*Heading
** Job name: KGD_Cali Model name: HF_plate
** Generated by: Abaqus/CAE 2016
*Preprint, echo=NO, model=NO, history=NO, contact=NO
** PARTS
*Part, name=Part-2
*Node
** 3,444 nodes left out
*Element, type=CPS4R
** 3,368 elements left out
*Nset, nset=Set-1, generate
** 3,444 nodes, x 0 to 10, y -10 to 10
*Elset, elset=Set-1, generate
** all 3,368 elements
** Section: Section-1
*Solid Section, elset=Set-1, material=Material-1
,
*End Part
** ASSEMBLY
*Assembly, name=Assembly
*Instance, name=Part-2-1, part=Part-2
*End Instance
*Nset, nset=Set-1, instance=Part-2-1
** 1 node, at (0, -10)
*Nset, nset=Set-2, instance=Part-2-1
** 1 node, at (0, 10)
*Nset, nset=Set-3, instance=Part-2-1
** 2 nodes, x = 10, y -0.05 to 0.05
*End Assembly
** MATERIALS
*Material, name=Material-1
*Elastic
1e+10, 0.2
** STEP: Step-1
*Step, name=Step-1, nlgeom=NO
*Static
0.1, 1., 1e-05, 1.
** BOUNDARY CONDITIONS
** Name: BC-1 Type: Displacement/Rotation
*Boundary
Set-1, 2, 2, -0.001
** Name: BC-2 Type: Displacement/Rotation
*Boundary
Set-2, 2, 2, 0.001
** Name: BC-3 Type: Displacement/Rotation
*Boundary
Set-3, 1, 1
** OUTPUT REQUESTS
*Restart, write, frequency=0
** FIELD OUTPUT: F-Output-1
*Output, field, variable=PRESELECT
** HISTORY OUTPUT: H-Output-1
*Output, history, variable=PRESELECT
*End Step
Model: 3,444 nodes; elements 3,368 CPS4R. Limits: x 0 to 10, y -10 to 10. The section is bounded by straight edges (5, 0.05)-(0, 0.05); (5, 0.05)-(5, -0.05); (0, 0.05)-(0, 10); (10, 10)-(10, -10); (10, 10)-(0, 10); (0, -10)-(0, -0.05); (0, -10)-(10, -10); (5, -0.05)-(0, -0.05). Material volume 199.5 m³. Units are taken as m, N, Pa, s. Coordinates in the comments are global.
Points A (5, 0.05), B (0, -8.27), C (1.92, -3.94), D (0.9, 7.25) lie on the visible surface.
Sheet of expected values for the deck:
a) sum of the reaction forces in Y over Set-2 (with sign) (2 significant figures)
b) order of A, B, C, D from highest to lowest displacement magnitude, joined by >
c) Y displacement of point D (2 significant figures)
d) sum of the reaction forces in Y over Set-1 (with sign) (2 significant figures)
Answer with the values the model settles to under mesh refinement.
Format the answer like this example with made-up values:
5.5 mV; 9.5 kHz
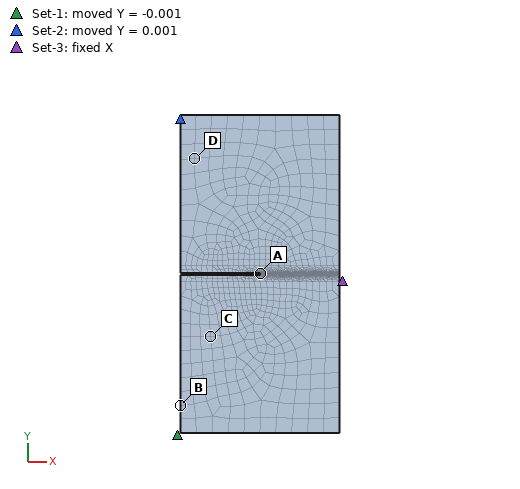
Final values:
4.3e+05 N; B > D > C > A; 6.1e-04 m; -4.3e+05 N
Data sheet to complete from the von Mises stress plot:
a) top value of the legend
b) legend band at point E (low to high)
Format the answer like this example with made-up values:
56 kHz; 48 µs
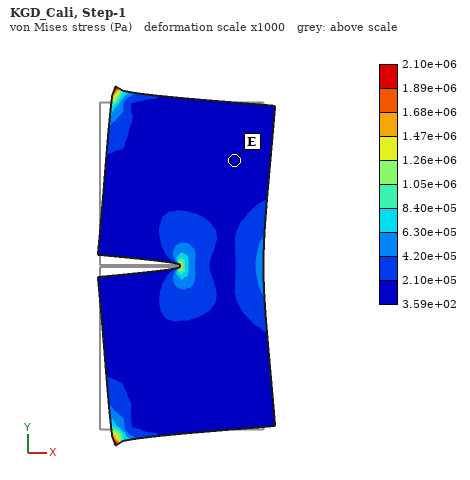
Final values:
2.10e+06 Pa; 3.59e+02 to 2.10e+05 Pa
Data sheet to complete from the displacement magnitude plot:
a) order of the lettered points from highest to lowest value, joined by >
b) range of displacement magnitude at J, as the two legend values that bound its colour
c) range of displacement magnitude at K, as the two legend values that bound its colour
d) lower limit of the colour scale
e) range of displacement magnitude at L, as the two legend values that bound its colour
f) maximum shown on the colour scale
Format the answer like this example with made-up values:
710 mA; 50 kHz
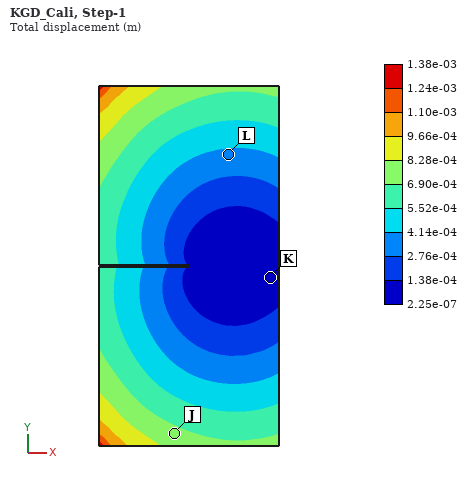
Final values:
J > L > K; 6.90e-04 to 8.28e-04 m; 2.25e-07 to 1.38e-04 m; 2.25e-07 m; 2.76e-04 to 4.14e-04 m; 1.38e-03 m
